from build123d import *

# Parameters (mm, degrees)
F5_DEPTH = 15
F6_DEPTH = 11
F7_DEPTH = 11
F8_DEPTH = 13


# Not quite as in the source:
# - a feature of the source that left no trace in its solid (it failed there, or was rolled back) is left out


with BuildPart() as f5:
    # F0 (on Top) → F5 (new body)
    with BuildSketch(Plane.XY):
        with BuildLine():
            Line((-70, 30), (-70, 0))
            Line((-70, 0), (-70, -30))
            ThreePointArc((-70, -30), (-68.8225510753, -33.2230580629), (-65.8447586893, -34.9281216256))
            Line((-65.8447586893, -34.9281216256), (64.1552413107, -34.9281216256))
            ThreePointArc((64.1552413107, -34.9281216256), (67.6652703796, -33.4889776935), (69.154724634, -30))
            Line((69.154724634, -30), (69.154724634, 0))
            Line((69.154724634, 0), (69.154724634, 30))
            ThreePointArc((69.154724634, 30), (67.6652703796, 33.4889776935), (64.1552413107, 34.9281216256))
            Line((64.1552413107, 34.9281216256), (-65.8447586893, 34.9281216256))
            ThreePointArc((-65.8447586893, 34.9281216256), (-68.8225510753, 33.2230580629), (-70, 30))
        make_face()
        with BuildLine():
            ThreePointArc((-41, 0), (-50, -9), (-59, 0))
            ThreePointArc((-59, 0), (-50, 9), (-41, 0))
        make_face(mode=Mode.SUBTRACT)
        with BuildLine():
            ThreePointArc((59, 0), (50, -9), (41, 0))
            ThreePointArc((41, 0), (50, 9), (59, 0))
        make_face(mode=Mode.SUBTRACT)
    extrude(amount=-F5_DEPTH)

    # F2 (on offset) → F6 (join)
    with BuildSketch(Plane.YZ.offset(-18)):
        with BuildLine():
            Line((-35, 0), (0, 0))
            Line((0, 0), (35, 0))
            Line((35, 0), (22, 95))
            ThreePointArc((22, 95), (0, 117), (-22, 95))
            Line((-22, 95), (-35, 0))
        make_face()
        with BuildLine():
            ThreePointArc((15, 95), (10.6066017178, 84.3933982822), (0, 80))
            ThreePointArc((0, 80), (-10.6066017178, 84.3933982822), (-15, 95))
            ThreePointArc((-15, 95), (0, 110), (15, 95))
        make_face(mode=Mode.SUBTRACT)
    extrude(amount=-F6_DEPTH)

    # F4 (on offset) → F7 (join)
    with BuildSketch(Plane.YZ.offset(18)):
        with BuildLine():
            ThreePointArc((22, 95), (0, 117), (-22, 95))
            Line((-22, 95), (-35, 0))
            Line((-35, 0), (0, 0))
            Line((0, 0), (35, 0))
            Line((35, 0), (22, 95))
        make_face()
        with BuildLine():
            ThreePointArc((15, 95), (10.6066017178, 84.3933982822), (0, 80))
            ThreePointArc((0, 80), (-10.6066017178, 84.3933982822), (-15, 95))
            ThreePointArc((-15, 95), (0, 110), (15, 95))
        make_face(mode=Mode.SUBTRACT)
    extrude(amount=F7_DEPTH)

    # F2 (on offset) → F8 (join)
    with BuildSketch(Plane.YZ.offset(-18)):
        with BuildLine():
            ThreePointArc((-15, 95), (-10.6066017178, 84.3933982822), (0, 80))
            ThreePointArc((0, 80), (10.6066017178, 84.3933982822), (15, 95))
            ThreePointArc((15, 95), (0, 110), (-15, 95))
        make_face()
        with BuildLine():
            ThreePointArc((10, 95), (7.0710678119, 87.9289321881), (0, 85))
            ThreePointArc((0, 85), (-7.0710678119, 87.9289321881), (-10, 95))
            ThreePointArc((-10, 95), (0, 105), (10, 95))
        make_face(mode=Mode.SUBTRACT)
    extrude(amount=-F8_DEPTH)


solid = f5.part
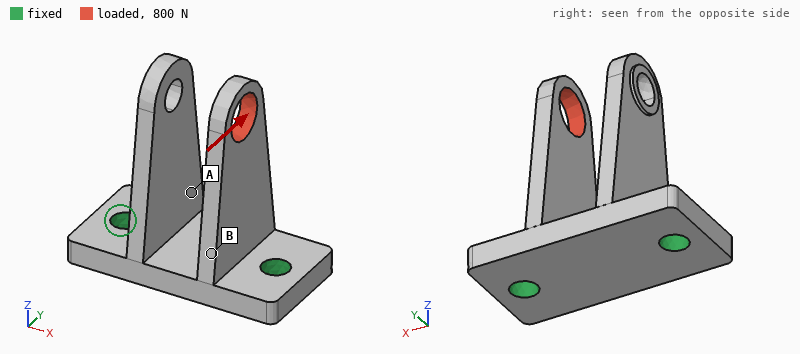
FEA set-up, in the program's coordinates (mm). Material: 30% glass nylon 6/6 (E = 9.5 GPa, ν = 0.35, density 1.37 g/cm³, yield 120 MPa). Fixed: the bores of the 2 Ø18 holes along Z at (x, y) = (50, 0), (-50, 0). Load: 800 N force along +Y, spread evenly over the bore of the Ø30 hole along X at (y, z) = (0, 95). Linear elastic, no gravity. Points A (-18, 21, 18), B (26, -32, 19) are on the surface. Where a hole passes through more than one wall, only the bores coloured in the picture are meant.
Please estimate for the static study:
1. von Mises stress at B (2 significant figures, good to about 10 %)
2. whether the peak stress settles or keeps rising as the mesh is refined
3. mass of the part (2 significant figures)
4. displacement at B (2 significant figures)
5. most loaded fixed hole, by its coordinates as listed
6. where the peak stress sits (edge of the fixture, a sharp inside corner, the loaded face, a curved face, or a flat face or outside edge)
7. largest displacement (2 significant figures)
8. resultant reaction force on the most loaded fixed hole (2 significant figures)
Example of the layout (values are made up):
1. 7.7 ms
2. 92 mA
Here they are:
1. 8.4 MPa
2. keeps rising
3. 360 g
4. 0.18 mm
5. (50, 0)
6. edge of the fixture
7. 0.73 mm
8. 620 N
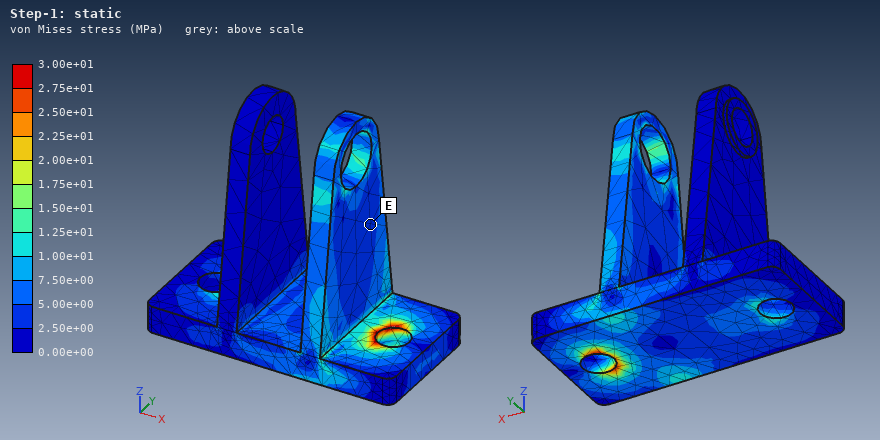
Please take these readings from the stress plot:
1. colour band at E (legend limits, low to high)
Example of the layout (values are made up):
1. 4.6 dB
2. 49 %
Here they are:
1. 2.50e+00 to 5.00e+00 MPa
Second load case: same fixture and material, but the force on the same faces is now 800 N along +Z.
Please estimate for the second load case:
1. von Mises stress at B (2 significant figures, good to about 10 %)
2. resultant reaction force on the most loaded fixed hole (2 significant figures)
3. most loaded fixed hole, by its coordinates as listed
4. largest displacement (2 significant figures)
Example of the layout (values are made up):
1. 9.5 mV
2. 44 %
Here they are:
1. 0.69 MPa
2. 660 N
3. (50, 0)
4. 65 µm
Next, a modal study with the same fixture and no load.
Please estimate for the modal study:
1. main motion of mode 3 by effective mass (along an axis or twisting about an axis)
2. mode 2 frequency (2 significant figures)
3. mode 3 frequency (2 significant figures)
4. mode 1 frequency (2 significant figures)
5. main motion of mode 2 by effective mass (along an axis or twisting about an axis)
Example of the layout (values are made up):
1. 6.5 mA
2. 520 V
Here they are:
1. along Y
2. 480 Hz
3. 890 Hz
4. 420 Hz
5. along X
